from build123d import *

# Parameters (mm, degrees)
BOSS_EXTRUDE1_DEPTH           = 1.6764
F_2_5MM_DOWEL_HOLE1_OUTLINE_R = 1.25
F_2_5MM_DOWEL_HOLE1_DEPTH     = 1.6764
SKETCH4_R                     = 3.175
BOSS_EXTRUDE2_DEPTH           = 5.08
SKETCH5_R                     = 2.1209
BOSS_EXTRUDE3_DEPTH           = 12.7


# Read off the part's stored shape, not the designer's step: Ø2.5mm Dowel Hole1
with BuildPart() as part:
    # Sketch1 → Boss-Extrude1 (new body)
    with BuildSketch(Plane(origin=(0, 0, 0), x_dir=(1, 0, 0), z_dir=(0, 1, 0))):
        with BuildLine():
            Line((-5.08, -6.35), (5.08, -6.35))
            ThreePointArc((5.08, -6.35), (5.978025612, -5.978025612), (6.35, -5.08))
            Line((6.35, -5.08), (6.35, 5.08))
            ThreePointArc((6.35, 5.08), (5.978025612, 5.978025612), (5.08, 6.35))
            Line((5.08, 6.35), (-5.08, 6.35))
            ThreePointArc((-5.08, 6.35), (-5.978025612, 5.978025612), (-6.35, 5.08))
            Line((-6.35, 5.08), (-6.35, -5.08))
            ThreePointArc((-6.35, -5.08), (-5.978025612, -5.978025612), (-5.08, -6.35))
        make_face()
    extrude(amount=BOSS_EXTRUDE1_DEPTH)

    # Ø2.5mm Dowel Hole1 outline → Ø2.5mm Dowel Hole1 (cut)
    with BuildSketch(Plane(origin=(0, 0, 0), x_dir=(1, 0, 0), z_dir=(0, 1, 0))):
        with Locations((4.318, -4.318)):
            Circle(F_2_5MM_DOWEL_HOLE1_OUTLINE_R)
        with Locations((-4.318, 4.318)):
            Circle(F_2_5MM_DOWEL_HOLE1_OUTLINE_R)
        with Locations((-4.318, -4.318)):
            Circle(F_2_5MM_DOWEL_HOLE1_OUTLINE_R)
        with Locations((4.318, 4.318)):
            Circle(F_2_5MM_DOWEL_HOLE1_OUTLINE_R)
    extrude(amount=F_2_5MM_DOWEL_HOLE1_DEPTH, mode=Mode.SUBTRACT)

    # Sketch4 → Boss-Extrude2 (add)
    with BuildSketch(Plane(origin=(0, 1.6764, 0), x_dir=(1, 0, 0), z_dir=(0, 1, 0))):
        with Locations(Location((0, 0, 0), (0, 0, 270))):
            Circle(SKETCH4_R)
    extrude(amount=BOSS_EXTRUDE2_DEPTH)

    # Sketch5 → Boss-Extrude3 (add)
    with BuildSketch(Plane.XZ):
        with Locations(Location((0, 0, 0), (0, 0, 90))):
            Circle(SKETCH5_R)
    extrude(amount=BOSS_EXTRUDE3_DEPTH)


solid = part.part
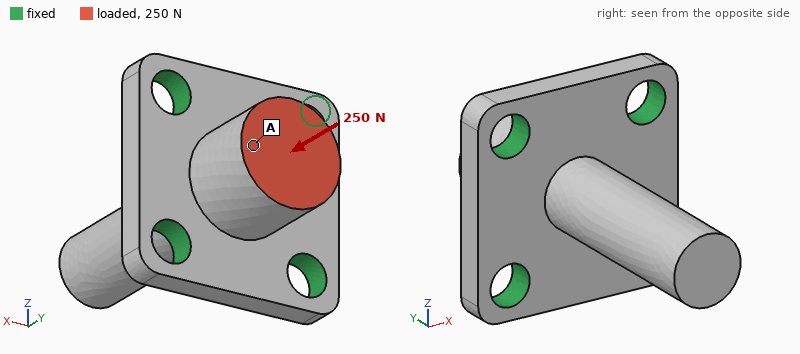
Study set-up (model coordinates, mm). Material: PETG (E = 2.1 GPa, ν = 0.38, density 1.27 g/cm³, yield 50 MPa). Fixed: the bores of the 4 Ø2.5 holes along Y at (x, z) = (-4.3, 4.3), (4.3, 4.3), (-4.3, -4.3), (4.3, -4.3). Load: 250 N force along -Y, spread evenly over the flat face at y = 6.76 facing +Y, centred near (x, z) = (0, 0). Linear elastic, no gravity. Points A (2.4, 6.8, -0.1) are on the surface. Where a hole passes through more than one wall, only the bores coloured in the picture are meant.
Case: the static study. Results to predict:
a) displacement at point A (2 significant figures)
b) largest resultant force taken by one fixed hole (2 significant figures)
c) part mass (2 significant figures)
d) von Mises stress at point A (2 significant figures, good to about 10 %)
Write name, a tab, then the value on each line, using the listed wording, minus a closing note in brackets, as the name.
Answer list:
displacement at point A	74 µm
largest resultant force taken by one fixed hole	65 N
part mass	0.73 g
von Mises stress at point A	8.0 MPa
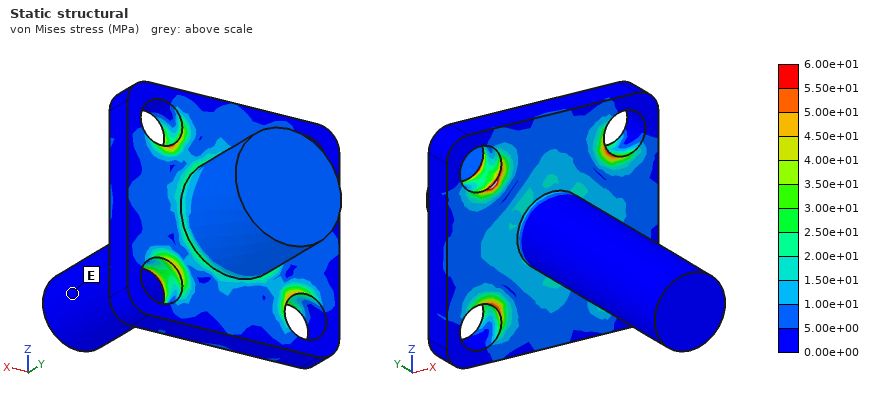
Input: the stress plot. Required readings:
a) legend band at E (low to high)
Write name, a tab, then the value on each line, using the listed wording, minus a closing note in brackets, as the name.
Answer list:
legend band at E	0.00e+00 to 5.00e+00 MPa
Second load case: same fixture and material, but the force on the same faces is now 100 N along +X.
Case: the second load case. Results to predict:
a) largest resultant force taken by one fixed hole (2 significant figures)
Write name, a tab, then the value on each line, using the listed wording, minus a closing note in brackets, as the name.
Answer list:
largest resultant force taken by one fixed hole	52 N
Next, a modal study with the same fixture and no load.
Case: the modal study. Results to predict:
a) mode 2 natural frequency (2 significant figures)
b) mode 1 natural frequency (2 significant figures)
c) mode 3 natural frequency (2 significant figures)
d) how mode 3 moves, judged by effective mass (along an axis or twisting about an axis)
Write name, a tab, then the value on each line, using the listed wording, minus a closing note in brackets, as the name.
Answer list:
mode 2 natural frequency	3600 Hz
mode 1 natural frequency	3600 Hz
mode 3 natural frequency	13 kHz
how mode 3 moves, judged by effective mass	along Y
